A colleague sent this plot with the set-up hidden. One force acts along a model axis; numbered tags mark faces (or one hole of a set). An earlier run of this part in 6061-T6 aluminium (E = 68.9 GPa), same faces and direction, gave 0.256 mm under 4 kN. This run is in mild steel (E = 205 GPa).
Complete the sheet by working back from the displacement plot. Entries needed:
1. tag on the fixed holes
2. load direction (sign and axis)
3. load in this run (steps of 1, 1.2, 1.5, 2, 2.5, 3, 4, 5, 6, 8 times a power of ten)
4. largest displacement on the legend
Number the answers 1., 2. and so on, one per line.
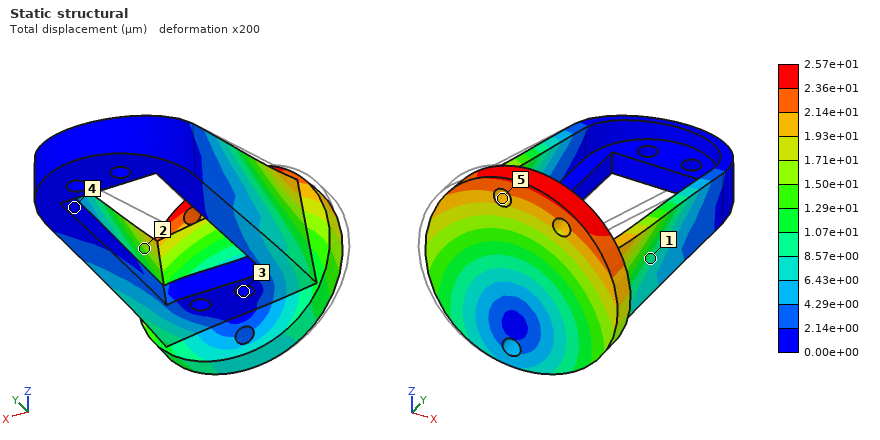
1. 3
2. +X
3. 1.2 kN
4. 2.57e+01 µm
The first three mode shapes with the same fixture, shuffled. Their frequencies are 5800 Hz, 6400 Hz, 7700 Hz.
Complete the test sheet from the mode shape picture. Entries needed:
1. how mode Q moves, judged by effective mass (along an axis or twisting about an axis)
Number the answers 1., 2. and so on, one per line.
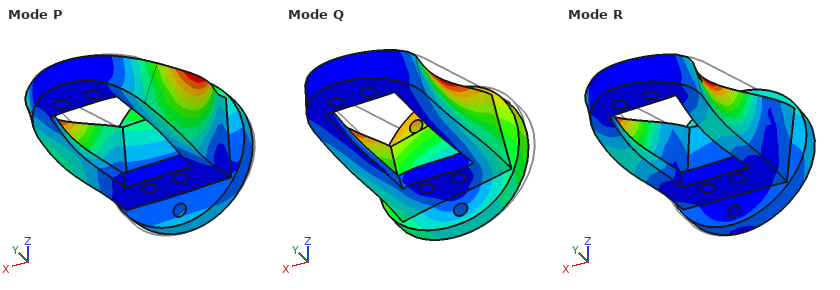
1. along X
